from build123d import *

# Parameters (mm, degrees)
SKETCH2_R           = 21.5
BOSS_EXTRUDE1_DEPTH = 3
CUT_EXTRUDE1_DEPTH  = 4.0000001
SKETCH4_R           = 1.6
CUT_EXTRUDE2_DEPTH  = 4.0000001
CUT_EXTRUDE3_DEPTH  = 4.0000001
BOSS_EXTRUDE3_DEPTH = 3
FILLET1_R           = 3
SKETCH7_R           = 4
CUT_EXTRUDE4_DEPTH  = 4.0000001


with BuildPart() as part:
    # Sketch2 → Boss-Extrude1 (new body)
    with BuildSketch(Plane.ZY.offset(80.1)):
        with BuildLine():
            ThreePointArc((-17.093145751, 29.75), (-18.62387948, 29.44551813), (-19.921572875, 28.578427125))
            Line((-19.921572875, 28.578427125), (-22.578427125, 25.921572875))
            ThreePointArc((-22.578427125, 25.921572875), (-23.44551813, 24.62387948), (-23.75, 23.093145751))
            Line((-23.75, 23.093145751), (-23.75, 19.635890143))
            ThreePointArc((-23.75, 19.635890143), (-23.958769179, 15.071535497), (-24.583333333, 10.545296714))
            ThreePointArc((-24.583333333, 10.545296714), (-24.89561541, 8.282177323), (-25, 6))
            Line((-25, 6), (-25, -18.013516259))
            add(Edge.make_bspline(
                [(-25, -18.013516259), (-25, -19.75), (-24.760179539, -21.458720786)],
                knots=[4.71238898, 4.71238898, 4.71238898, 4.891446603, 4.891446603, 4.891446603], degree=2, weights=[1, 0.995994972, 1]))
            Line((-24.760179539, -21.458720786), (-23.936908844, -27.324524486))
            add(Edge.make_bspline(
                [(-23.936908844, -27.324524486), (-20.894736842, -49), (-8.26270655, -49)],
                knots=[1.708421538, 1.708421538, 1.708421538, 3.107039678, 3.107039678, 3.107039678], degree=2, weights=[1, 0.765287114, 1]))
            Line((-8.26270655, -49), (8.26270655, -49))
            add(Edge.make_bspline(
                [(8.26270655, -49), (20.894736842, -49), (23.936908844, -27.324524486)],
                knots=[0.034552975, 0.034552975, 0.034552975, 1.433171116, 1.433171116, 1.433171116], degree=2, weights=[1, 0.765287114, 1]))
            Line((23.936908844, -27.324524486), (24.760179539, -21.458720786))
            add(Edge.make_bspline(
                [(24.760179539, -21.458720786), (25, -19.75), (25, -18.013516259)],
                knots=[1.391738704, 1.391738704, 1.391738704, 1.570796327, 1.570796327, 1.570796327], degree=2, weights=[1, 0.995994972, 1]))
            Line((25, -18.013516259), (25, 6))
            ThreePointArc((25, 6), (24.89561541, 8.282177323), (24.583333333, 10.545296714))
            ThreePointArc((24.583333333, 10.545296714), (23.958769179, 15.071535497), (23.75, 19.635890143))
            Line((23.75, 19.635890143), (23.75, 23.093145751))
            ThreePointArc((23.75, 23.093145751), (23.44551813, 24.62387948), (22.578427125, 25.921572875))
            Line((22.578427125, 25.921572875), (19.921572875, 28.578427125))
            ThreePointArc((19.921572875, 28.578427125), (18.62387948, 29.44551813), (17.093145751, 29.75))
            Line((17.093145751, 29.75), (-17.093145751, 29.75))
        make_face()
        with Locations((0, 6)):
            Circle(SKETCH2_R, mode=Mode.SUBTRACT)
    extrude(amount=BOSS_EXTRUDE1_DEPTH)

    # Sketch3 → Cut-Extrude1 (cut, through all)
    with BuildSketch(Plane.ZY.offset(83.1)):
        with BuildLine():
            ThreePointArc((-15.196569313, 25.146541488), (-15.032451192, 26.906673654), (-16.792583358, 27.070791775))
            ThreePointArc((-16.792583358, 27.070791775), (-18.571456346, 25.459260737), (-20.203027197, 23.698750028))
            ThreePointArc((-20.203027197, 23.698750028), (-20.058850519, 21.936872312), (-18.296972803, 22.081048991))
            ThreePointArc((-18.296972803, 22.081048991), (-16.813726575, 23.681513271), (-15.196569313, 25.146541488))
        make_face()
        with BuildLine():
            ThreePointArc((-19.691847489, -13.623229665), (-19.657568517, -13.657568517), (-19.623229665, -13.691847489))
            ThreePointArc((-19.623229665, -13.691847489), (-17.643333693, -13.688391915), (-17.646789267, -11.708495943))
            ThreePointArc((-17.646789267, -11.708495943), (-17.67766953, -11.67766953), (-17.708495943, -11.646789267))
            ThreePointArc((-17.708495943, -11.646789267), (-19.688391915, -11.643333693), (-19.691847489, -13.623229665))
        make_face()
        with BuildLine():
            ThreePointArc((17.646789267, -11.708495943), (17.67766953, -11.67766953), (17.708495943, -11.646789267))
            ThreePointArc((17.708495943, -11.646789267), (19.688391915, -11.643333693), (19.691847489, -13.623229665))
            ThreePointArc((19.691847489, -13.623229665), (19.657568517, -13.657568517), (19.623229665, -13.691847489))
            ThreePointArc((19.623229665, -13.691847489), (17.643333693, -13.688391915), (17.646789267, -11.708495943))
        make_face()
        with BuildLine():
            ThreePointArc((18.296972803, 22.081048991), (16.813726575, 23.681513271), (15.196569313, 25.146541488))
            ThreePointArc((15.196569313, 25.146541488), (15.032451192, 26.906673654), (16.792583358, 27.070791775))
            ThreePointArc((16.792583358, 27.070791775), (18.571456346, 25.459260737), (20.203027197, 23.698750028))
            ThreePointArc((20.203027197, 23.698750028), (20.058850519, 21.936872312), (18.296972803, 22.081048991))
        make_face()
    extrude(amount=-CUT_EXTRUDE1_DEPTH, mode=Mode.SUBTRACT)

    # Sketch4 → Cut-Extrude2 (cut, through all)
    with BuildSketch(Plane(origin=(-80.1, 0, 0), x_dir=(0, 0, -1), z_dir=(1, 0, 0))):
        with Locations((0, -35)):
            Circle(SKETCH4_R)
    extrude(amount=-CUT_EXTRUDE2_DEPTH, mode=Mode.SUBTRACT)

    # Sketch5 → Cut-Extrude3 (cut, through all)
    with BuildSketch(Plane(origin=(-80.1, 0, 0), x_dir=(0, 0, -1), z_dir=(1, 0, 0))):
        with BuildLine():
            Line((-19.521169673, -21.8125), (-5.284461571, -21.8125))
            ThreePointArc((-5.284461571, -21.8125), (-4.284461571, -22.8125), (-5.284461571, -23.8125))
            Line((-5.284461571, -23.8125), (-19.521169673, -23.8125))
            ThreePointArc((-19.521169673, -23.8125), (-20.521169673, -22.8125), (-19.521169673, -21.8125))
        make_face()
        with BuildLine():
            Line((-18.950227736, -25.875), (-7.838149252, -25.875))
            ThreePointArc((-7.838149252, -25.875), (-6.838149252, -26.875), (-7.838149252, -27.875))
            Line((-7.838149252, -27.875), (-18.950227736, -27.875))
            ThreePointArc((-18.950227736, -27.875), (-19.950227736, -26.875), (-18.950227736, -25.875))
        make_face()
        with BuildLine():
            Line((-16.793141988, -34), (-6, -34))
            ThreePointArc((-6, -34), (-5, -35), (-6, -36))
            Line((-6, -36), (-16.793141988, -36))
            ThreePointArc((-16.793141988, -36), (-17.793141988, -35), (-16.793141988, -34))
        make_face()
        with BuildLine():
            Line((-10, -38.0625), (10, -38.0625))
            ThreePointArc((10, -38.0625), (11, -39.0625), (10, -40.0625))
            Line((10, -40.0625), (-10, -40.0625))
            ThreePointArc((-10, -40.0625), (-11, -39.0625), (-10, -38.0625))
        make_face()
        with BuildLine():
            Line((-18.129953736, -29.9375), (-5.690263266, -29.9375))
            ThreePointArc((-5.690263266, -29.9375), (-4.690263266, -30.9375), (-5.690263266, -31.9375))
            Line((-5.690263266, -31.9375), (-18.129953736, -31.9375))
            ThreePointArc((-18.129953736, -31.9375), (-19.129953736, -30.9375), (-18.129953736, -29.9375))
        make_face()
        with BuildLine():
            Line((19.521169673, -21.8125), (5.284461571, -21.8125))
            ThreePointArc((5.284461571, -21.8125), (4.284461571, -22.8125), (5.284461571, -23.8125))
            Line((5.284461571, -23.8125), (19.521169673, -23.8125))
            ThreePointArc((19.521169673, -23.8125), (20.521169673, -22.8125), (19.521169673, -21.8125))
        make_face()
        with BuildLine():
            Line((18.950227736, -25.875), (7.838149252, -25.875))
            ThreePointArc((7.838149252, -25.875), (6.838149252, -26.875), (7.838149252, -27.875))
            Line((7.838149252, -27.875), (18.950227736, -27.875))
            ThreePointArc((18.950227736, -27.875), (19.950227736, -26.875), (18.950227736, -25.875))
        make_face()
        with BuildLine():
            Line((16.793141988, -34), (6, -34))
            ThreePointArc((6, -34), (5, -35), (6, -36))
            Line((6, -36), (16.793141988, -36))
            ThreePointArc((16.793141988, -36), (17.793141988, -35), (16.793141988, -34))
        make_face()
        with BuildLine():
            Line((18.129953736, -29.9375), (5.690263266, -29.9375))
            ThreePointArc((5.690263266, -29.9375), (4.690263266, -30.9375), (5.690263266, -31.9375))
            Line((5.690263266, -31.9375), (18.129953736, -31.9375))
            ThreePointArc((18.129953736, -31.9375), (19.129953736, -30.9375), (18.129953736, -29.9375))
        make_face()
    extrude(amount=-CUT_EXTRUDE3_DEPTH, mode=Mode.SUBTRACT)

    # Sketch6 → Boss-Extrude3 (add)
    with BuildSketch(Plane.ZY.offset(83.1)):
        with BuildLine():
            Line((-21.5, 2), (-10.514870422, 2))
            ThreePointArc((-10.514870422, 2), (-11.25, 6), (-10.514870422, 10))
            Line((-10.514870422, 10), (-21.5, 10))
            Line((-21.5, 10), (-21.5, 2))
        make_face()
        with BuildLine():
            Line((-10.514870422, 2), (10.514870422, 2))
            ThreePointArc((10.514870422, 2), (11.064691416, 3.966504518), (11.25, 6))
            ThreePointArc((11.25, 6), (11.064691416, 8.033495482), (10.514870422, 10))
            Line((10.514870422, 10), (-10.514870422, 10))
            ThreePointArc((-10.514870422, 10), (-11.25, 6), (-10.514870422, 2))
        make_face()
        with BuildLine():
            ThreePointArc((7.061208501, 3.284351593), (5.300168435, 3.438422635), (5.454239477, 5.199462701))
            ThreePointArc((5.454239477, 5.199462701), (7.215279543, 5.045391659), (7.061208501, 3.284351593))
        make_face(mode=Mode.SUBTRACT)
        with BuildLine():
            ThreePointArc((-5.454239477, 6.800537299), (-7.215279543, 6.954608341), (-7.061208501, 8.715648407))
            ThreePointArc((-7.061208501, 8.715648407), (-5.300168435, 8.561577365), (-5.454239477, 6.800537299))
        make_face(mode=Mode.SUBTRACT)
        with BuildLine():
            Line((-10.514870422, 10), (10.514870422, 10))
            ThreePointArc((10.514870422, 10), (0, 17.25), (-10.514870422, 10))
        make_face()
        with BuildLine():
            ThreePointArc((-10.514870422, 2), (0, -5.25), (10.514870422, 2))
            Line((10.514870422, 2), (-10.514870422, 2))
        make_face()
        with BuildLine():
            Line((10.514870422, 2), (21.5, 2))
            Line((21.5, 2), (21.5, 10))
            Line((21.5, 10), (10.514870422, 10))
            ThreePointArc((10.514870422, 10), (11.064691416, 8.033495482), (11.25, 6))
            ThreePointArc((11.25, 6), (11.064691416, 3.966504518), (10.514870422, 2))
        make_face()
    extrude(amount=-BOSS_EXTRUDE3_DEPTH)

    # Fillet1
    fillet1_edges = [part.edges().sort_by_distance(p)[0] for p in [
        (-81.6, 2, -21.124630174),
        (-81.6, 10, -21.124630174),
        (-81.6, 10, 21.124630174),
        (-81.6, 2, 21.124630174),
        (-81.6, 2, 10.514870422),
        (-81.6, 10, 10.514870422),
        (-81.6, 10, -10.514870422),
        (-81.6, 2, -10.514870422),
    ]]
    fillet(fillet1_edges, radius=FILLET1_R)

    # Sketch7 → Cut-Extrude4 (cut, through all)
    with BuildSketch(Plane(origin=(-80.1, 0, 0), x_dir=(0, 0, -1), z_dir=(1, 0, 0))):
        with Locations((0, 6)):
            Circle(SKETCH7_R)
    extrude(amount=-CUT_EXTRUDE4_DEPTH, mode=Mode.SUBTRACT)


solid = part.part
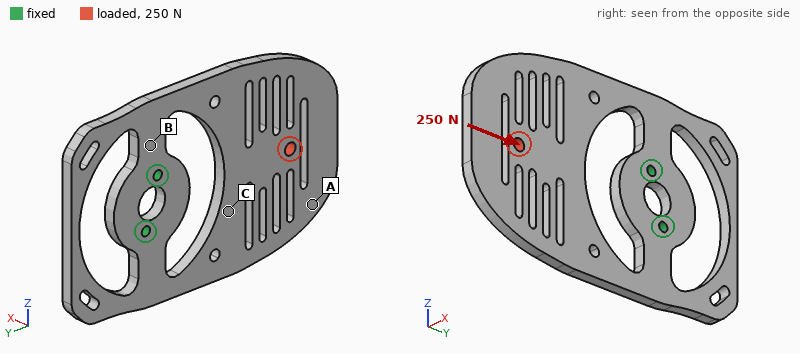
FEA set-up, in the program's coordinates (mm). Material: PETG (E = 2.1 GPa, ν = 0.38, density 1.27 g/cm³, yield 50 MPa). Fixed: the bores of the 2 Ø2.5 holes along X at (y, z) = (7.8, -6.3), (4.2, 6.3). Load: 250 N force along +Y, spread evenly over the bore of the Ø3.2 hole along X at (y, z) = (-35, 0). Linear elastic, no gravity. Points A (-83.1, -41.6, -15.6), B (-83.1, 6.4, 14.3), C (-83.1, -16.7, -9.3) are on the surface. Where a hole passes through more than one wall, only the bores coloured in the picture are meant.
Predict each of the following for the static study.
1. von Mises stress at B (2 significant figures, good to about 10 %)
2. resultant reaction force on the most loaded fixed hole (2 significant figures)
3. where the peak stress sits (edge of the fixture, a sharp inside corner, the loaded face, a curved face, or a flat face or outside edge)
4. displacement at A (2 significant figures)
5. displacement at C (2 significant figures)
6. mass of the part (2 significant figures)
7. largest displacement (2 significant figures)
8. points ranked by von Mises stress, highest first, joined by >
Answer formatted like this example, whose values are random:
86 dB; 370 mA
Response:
13 MPa; 130 N; a curved face; 0.48 mm; 0.65 mm; 9.1 g; 0.84 mm; B > C > A
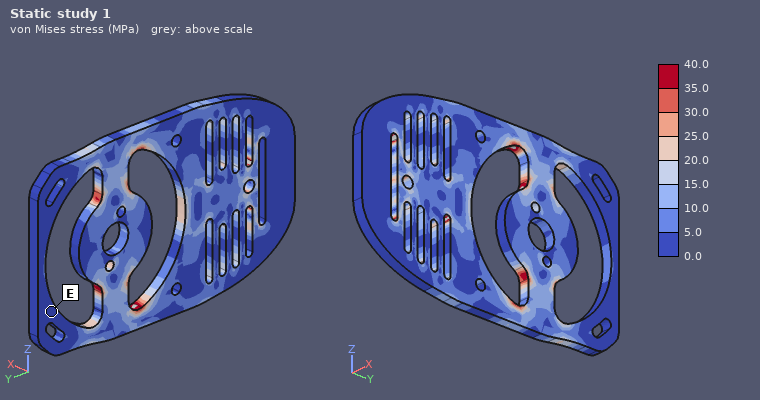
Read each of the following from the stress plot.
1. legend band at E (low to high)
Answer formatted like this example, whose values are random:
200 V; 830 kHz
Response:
0.0 to 5.0 MPa
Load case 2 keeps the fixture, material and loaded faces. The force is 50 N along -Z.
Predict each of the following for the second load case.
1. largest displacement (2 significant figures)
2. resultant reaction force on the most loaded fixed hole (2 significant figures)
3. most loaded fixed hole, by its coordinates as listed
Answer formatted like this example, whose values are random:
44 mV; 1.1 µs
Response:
0.96 mm; 140 N; (4.2, 6.3)
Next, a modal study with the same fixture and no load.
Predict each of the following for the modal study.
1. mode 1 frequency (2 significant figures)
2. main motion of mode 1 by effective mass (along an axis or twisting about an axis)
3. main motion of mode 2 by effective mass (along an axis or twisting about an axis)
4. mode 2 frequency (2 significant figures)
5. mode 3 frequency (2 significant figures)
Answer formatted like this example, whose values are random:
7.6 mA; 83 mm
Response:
100 Hz; along X; twisting about Y; 400 Hz; 510 Hz
